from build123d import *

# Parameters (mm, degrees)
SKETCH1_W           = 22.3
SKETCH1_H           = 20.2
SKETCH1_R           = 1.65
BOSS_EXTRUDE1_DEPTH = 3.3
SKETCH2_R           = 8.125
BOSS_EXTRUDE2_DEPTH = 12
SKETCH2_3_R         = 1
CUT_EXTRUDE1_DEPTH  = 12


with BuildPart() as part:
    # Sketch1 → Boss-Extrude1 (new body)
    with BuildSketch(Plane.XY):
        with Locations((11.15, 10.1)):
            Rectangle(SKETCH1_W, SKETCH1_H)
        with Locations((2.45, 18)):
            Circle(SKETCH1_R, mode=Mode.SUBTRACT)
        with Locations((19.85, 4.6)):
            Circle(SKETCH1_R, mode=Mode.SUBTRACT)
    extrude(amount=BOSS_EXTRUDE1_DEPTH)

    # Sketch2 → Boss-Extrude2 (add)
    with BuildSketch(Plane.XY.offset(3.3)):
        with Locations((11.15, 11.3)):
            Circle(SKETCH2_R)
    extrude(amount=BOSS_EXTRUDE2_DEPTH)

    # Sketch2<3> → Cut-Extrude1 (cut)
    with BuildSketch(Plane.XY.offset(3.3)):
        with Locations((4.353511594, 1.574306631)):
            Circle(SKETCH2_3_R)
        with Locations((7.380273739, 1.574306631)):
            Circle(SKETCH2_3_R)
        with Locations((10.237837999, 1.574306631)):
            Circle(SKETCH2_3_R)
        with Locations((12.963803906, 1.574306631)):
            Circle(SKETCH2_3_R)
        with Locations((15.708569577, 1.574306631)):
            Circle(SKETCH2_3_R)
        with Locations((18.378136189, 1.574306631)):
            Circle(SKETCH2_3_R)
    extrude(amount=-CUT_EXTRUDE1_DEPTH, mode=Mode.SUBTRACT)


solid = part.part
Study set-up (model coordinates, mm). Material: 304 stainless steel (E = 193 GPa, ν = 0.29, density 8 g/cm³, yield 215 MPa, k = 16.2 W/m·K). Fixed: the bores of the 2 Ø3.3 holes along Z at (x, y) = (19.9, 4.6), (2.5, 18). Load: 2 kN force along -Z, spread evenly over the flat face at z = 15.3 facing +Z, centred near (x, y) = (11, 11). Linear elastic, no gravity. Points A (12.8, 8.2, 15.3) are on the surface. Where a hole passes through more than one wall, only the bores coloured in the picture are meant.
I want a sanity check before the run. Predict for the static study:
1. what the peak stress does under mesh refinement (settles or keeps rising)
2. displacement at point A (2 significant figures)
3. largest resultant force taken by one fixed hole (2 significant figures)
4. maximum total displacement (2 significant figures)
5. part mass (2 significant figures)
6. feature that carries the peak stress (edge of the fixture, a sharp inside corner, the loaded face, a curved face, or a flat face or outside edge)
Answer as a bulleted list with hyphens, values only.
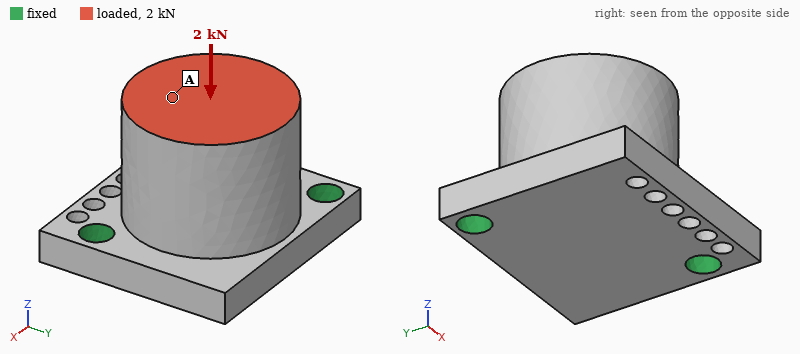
- keeps rising
- 3.8 µm
- 1.1 kN
- 4.3 µm
- 31 g
- edge of the fixture
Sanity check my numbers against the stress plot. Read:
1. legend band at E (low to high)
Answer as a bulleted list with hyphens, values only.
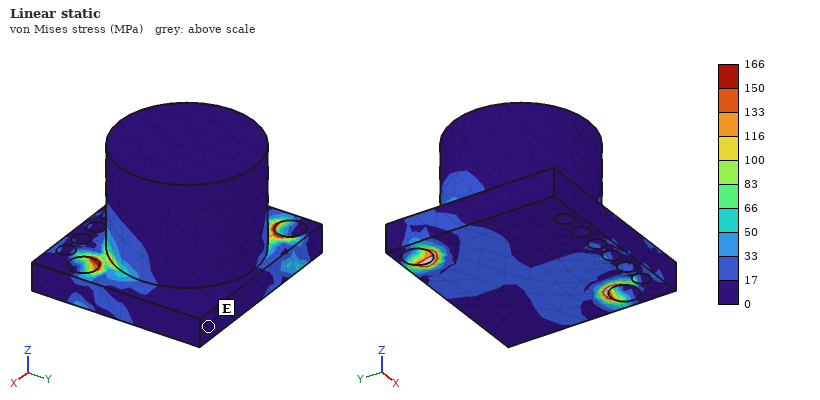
- 0 to 17 MPa
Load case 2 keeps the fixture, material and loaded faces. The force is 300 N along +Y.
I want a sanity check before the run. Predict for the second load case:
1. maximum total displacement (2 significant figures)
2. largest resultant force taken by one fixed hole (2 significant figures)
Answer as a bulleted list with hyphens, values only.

- 12 µm
- 210 N
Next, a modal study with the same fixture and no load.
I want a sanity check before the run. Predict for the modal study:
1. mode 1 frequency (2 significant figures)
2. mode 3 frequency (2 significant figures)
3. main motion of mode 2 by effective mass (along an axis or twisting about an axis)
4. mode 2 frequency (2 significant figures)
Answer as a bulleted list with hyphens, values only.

- 7400 Hz
- 23 kHz
- along Z
- 22 kHz
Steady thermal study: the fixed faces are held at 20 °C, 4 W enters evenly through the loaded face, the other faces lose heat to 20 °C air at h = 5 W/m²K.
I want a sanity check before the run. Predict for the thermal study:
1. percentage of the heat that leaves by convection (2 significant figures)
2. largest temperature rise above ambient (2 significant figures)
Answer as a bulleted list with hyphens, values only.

- 3.5 %
- 32 K
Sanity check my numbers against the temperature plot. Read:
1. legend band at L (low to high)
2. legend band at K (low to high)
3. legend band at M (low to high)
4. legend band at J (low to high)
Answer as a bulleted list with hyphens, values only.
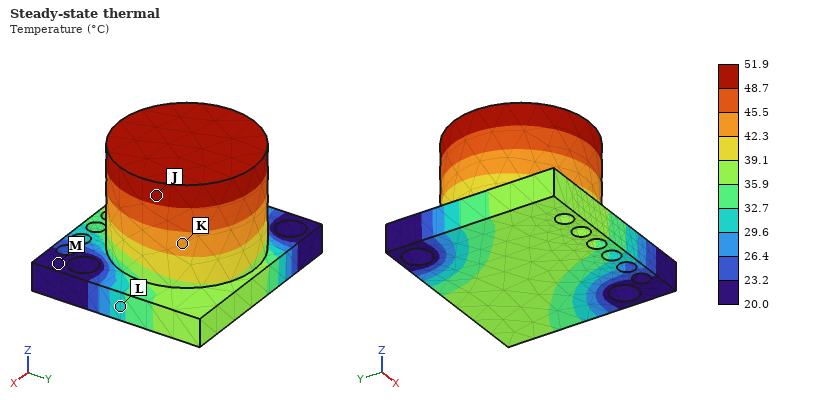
- 29.6 to 32.7 °C
- 42.3 to 45.5 °C
- 20.0 to 23.2 °C
- 48.7 to 51.9 °C
